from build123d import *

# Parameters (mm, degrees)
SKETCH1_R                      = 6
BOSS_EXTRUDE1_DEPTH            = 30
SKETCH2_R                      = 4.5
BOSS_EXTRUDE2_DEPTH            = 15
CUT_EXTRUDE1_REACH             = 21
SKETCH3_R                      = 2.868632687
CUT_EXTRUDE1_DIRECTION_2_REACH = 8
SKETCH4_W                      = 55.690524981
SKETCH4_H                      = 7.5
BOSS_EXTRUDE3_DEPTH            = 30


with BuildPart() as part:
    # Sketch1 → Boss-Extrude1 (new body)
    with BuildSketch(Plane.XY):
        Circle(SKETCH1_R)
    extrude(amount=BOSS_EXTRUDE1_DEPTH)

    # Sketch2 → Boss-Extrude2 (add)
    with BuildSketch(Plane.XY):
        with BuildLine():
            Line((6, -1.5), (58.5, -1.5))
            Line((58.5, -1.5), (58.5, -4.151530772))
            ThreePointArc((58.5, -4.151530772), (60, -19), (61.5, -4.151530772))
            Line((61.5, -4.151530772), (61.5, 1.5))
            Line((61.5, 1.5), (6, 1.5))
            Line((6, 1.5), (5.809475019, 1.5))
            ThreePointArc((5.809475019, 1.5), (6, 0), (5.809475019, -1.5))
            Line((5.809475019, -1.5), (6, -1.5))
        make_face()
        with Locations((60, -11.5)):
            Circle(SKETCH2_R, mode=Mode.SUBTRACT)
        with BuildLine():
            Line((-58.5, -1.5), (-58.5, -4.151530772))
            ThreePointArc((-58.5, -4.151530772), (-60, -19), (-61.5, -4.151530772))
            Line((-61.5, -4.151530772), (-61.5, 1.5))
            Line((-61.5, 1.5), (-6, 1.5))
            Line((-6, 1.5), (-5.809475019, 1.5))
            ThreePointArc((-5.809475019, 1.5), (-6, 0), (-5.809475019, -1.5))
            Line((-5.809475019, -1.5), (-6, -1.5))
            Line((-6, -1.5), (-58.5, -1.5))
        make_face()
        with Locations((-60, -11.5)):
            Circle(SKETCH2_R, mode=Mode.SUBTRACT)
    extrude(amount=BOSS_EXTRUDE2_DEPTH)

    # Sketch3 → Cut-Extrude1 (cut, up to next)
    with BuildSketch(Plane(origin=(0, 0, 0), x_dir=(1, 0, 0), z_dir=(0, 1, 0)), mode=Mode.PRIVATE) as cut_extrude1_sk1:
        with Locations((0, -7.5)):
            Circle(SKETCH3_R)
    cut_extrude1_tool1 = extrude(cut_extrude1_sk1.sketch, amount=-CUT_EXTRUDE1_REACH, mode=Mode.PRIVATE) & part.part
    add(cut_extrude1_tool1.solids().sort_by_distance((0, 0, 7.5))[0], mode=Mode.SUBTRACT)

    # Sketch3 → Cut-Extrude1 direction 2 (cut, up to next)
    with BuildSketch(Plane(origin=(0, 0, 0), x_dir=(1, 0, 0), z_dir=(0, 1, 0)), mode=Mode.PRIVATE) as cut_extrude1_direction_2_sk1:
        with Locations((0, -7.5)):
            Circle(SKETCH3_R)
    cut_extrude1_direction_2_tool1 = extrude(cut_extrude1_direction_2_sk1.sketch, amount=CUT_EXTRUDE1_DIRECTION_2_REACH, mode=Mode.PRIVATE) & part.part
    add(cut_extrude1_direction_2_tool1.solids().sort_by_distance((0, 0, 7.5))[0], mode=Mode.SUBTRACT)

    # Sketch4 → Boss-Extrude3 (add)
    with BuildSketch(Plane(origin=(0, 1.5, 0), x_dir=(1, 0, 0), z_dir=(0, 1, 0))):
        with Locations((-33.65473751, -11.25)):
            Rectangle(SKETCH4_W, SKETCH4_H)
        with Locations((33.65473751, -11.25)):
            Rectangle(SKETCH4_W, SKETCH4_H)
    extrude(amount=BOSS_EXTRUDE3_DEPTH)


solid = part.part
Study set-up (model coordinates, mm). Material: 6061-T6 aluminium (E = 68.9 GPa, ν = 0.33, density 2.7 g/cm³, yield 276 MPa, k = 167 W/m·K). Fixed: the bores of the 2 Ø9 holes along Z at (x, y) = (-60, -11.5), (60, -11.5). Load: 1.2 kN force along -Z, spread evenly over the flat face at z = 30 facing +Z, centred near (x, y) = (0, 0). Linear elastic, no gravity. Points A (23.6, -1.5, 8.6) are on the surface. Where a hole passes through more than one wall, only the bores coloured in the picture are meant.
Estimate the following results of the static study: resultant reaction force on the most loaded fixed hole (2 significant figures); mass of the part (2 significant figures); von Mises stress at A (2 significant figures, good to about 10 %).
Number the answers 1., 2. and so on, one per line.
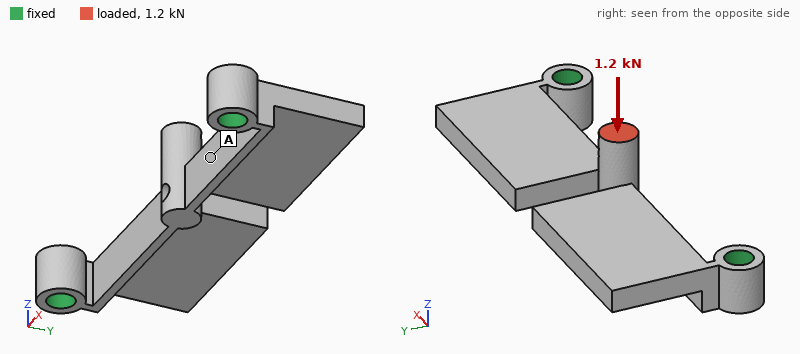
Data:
1. 610 N
2. 99 g
3. 29 MPa
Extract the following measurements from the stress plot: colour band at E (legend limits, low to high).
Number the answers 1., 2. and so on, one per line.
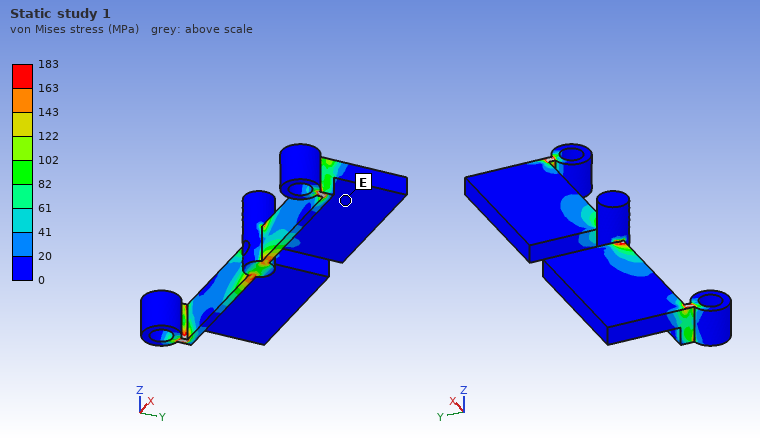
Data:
1. 0 to 20 MPa
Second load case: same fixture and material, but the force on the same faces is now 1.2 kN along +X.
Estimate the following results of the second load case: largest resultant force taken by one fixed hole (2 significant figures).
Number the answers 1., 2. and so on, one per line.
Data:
1. 650 N
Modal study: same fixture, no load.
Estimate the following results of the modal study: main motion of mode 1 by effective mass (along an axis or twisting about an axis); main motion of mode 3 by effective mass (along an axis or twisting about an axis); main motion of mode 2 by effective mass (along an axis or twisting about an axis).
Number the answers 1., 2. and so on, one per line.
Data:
1. along Y
2. twisting about Y
3. along Z
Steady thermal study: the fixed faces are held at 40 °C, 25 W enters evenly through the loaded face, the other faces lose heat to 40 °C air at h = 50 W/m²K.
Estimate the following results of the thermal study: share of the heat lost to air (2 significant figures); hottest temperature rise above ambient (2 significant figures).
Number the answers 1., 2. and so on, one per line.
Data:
1. 43 %
2. 55 K
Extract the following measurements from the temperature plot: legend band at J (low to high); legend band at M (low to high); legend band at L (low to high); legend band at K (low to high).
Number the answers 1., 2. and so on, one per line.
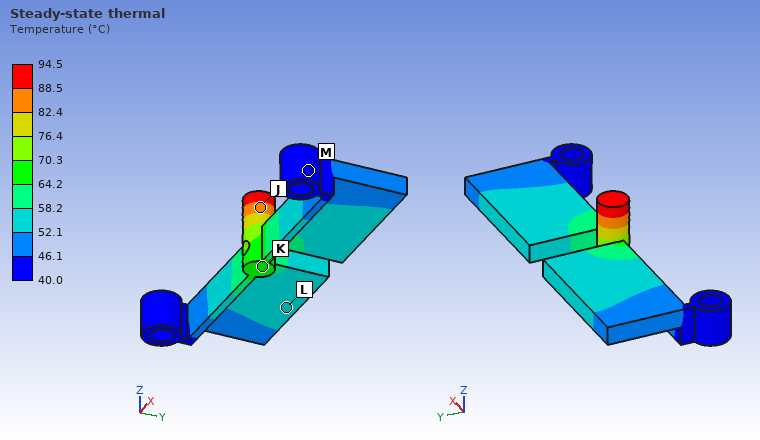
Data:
1. 82.4 to 88.5 °C
2. 40.0 to 46.1 °C
3. 52.1 to 58.2 °C
4. 64.2 to 70.3 °C
